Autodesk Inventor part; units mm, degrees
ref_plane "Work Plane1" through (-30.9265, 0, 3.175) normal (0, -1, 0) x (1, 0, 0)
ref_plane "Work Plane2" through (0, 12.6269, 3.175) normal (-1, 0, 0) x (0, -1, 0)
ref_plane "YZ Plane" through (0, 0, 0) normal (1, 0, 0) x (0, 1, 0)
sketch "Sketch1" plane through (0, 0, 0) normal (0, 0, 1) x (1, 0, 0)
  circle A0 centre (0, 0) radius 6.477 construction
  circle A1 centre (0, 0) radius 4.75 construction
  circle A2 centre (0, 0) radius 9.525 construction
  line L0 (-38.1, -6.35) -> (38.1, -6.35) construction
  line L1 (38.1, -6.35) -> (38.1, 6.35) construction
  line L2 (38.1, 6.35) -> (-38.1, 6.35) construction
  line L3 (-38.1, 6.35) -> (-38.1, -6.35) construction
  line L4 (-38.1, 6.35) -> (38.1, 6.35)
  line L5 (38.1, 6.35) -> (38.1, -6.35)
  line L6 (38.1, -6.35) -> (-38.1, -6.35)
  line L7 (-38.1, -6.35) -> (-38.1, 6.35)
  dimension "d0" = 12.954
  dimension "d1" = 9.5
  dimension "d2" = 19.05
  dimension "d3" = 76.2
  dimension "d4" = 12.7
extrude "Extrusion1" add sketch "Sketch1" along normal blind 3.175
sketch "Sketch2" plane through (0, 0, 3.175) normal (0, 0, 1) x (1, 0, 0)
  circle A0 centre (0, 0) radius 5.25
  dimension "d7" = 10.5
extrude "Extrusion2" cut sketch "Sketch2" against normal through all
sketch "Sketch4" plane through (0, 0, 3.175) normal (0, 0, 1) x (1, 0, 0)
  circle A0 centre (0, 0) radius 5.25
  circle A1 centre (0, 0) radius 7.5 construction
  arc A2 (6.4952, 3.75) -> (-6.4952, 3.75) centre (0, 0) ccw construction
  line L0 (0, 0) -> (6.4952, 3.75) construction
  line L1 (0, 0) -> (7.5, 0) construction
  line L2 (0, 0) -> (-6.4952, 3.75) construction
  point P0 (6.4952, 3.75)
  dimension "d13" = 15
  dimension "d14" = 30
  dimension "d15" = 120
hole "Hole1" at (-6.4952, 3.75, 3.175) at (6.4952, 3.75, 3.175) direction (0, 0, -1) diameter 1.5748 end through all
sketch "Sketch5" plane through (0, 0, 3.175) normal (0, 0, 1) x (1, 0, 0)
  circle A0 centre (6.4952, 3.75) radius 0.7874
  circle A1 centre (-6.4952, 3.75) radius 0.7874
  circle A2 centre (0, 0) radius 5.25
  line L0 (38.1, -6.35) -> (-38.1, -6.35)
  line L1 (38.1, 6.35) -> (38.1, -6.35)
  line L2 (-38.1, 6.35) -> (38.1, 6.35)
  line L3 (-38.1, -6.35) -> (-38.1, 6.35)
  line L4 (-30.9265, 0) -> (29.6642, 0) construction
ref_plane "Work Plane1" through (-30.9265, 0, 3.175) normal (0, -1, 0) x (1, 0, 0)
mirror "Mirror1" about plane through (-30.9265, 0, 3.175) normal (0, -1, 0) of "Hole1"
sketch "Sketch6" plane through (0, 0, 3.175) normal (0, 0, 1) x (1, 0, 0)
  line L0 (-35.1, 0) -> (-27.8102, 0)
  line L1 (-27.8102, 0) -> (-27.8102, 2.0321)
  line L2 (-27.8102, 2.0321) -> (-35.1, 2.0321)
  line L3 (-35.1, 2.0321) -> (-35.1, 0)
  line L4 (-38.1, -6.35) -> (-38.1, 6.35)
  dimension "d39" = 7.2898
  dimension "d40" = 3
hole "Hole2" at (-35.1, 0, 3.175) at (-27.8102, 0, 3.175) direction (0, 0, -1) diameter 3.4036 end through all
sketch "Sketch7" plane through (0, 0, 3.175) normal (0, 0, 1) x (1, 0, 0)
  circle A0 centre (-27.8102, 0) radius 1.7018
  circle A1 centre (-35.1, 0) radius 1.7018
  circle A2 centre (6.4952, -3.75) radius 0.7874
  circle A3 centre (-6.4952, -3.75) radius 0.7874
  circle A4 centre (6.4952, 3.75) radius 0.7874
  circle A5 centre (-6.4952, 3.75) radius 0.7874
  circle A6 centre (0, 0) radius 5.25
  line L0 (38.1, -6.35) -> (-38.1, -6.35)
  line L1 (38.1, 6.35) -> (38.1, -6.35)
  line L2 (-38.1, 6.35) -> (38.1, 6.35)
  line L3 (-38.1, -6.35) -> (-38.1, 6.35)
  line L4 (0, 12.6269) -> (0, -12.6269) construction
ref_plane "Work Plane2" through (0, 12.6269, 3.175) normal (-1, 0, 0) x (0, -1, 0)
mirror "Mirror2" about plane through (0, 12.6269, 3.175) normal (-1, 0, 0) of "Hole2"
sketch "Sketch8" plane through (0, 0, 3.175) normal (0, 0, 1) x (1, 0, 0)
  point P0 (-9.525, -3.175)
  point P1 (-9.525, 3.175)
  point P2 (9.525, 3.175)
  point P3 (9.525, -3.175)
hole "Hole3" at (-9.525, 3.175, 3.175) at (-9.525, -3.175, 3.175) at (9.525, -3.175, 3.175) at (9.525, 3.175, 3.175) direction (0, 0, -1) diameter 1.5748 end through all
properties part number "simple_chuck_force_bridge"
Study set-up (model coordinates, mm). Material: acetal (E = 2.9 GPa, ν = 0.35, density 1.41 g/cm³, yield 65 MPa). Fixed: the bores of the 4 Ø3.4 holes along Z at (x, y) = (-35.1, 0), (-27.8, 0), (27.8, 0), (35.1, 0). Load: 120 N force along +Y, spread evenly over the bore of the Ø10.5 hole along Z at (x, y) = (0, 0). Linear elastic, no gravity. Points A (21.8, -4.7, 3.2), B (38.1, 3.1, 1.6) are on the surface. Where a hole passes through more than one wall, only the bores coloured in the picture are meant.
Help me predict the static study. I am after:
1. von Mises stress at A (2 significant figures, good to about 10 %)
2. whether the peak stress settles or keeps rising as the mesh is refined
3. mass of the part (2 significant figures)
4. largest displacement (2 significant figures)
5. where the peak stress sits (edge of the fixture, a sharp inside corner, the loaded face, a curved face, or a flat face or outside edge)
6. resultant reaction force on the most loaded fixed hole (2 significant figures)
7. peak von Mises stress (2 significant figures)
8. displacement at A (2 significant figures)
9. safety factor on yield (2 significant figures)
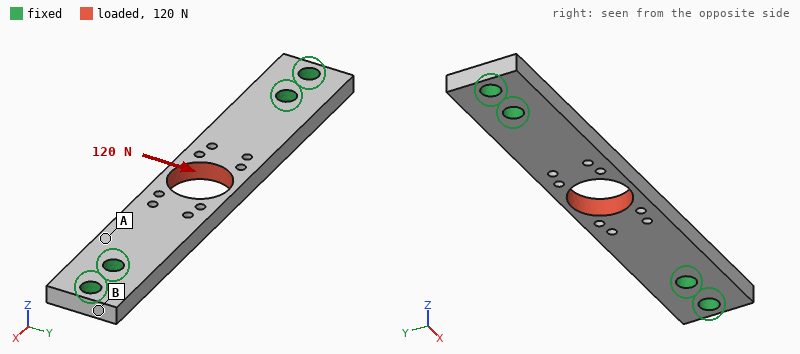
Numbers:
4.3 MPa
settles
3.7 g
0.16 mm
the loaded face
110 N
18 MPa
0.036 mm
3.6
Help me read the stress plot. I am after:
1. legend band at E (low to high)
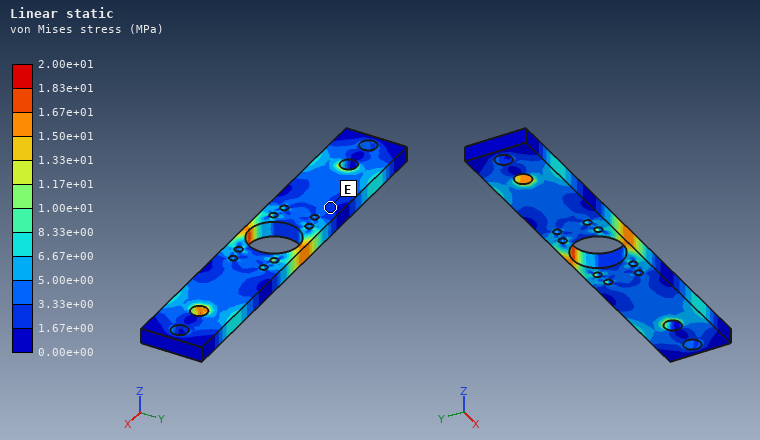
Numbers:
1.67e+00 to 3.33e+00 MPa
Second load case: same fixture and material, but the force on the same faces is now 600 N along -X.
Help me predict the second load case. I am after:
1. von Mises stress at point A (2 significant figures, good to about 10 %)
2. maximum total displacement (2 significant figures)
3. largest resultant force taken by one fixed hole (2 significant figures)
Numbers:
6.6 MPa
86 µm
250 N
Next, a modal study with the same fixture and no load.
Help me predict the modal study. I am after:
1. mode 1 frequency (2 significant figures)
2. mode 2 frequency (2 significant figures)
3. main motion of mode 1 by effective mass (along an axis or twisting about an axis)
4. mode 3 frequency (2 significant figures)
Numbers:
1600 Hz
3800 Hz
along Z
3900 Hz
